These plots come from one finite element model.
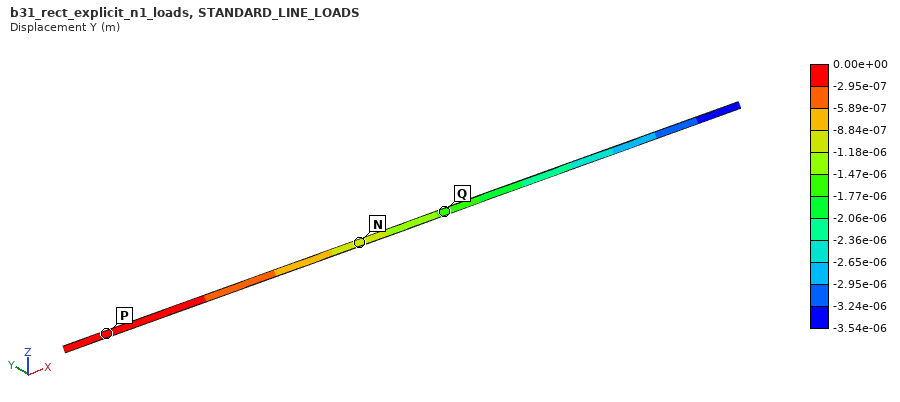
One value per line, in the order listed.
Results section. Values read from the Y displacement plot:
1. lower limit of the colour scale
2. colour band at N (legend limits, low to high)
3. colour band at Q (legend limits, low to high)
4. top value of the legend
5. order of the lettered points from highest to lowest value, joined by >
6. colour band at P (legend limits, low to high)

-3.54e-06 m
-1.18e-06 to -8.84e-07 m
-1.77e-06 to -1.47e-06 m
0.00e+00 m
P > N > Q
-2.95e-07 to 0.00e+00 m
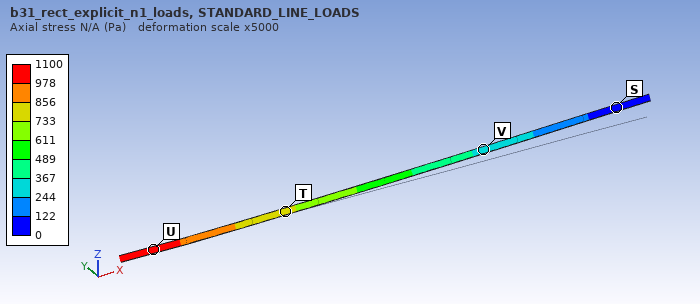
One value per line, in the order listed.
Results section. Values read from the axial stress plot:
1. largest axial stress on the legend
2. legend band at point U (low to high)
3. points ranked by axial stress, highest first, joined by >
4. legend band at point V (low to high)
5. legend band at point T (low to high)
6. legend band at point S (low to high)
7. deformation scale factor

1100 Pa
978 to 1100 Pa
U > T > V > S
244 to 367 Pa
733 to 856 Pa
0 to 122 Pa
5000
